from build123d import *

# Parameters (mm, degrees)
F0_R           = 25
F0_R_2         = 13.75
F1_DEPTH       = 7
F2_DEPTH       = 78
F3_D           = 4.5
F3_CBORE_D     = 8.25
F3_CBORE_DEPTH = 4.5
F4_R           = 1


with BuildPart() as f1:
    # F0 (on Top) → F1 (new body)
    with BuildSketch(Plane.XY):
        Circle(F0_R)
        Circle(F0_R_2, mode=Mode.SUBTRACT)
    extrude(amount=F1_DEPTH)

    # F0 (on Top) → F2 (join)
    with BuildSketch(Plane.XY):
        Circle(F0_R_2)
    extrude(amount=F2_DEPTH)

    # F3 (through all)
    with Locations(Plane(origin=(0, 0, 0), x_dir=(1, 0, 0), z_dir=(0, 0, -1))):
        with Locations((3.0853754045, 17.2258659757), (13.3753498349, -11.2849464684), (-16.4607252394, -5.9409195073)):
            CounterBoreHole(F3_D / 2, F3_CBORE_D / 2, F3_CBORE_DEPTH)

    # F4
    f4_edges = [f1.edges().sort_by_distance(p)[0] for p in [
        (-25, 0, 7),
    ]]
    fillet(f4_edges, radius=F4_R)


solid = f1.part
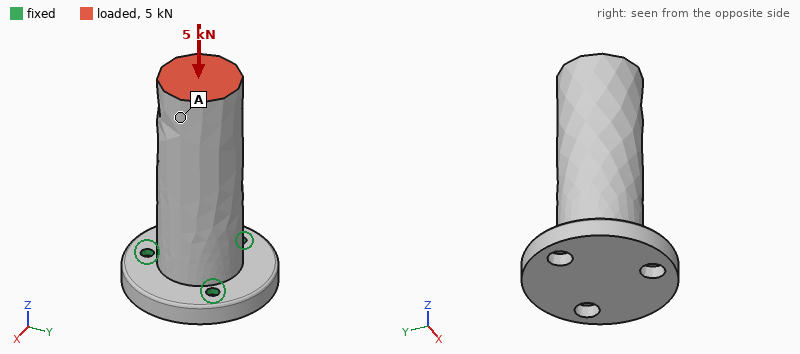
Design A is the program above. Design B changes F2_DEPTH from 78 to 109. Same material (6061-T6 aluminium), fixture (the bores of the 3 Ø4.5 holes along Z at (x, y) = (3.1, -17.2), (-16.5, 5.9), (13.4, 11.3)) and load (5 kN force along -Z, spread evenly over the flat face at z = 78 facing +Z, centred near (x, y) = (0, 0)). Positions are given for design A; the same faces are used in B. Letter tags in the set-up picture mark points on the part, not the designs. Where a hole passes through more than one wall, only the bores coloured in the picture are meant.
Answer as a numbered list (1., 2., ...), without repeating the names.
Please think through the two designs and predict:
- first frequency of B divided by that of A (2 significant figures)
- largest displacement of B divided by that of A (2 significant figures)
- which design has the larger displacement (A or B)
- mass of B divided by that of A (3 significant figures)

1. 0.55
2. 1.2
3. B
4. 1.33
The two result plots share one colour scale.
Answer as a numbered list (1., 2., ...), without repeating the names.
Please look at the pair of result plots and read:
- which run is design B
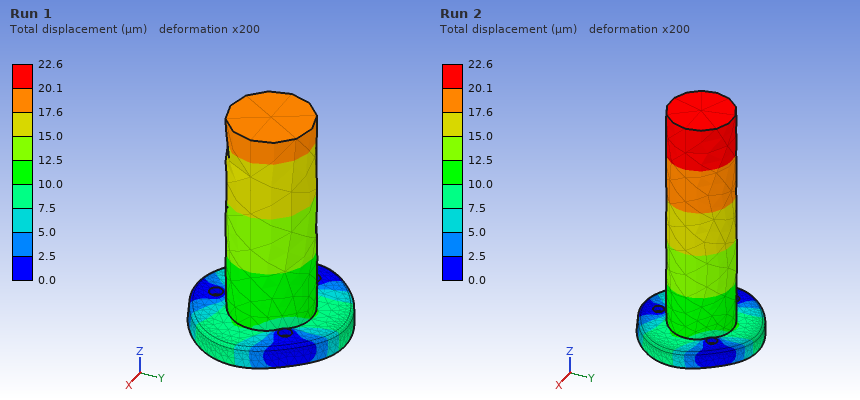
1. Run 2
